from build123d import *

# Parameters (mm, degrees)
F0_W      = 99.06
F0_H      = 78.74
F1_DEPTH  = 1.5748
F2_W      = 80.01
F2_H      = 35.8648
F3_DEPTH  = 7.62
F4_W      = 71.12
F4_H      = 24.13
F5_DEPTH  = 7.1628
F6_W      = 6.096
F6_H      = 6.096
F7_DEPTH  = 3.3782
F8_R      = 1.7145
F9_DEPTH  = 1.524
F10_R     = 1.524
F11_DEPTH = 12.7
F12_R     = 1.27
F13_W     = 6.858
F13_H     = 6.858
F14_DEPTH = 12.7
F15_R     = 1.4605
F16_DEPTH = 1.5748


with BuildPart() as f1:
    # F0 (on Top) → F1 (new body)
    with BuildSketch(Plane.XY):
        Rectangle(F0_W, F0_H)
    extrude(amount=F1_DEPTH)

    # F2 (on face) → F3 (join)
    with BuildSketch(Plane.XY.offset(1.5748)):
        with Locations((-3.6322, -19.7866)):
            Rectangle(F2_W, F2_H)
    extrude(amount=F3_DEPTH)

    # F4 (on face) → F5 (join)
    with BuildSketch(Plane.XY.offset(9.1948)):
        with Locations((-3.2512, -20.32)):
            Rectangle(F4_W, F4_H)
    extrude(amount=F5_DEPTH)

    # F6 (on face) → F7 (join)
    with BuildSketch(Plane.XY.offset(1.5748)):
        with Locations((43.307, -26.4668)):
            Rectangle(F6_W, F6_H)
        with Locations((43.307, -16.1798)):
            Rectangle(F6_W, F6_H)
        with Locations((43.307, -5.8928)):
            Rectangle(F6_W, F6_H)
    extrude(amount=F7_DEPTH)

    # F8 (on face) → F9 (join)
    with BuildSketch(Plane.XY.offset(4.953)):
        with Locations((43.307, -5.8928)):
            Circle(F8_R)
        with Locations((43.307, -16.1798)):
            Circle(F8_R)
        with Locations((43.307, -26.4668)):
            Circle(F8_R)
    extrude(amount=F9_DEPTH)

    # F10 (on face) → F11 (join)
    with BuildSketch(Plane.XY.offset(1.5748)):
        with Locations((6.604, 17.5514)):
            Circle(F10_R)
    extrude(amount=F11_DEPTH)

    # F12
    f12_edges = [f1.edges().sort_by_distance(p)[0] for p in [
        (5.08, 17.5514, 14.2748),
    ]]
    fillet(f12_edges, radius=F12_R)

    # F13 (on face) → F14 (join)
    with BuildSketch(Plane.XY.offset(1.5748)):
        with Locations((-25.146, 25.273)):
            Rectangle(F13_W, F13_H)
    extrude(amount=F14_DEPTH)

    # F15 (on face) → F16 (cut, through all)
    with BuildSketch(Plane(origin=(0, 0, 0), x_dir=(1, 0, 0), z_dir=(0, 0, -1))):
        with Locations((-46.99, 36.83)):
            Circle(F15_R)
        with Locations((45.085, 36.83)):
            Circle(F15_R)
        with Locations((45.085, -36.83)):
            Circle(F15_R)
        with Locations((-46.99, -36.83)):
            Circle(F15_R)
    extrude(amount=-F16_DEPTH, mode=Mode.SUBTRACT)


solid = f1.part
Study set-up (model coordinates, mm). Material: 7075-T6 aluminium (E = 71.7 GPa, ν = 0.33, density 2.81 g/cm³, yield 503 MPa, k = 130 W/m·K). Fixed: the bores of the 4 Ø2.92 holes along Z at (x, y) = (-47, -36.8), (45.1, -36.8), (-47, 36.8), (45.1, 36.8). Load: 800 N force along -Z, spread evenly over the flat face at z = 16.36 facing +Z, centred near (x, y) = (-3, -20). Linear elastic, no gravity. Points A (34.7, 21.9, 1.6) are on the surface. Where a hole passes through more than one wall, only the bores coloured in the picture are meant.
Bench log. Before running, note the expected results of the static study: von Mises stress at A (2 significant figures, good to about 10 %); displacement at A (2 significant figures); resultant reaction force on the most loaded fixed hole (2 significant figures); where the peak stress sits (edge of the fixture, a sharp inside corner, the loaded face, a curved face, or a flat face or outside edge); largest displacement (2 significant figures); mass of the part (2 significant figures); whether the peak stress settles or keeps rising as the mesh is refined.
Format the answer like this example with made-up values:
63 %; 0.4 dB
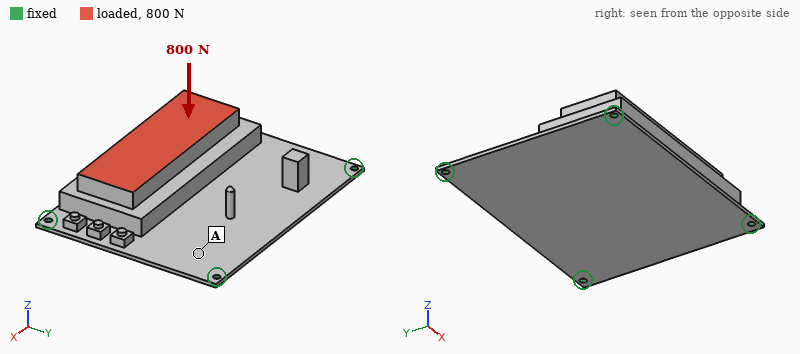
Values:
24 MPa; 0.26 mm; 420 N; edge of the fixture; 0.49 mm; 130 g; keeps rising
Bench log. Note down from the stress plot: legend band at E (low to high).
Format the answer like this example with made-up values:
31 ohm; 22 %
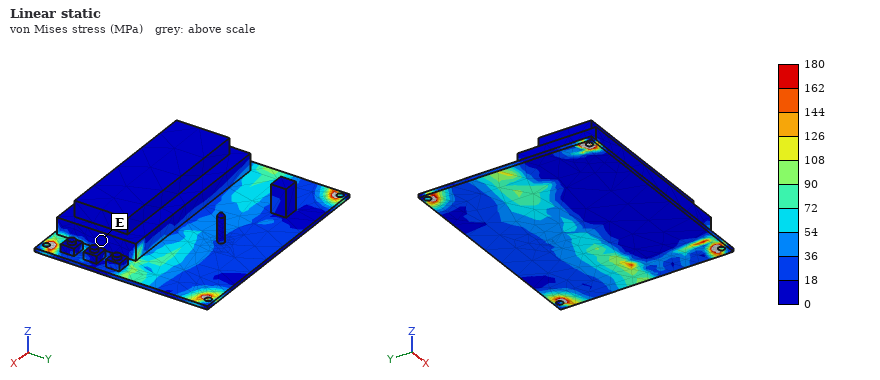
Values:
0 to 18 MPa
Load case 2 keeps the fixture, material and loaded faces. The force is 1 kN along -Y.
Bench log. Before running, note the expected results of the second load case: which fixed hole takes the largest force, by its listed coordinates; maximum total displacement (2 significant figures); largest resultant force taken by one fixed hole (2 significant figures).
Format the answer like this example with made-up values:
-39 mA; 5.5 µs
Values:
(-47, -36.8); 0.59 mm; 420 N
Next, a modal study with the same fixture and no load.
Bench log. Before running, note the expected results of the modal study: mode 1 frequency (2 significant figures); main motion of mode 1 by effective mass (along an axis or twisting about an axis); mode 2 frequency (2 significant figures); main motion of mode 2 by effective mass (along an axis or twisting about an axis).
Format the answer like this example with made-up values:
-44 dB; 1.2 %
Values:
630 Hz; along Z; 1500 Hz; twisting about X
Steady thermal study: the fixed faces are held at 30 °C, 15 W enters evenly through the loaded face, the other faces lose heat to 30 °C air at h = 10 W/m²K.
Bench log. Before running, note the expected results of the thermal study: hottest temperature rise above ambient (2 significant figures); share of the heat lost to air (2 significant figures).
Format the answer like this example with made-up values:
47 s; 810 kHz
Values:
17 K; 16 %
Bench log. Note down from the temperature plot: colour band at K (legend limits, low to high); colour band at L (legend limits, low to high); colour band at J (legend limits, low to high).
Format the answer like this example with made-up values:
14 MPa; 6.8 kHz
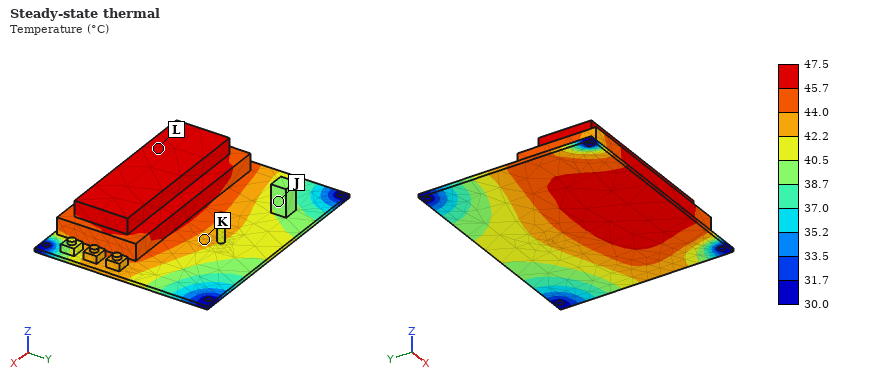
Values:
42.2 to 44.0 °C; 45.7 to 47.5 °C; 38.7 to 40.5 °C
